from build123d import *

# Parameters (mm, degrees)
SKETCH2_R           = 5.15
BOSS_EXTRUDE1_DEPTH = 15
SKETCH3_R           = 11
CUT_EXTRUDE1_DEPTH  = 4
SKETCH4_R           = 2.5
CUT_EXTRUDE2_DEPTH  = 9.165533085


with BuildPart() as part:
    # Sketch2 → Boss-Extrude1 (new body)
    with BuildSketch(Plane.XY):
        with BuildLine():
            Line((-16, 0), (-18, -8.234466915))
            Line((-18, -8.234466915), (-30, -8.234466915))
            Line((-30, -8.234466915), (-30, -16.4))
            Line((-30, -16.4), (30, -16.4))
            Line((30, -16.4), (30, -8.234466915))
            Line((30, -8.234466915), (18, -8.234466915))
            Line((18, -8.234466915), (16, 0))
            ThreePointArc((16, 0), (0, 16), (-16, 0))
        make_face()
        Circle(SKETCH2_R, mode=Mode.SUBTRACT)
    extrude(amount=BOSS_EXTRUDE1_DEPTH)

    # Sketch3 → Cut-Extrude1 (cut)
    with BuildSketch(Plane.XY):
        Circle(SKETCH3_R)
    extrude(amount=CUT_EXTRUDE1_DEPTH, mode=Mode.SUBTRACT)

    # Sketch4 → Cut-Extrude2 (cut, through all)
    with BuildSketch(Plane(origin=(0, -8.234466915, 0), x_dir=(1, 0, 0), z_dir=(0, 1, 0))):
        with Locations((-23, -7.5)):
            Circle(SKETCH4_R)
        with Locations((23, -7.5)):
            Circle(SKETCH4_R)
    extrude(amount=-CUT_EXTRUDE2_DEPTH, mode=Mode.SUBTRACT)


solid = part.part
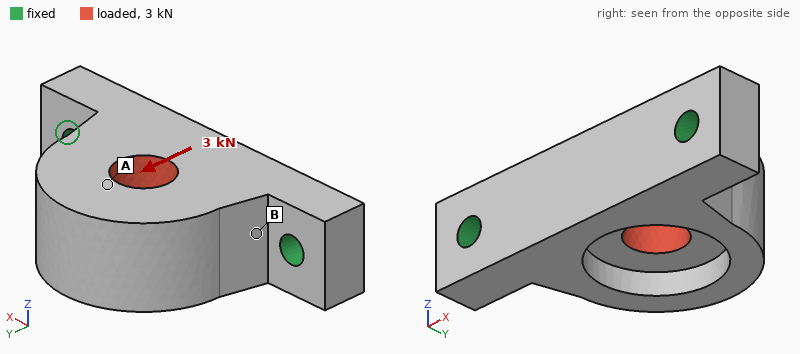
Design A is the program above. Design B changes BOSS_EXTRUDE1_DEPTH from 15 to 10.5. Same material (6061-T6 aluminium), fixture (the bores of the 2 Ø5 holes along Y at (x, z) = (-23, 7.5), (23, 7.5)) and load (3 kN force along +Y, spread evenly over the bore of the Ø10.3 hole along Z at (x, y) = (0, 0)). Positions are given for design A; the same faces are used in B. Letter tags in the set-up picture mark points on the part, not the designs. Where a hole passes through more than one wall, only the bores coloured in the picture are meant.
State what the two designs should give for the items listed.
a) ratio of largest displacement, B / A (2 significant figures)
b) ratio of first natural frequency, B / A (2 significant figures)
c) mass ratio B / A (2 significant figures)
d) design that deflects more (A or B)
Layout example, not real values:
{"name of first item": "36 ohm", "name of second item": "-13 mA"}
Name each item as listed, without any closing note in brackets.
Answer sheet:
{"ratio of largest displacement, B / A": "1.4", "ratio of first natural frequency, B / A": "0.88", "mass ratio B / A": "0.67", "design that deflects more": "B"}
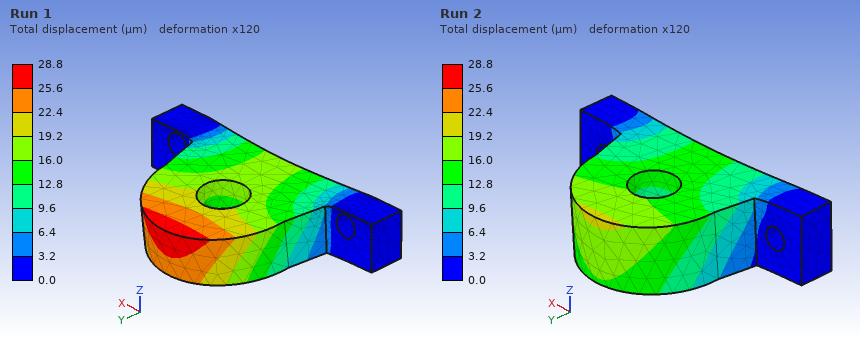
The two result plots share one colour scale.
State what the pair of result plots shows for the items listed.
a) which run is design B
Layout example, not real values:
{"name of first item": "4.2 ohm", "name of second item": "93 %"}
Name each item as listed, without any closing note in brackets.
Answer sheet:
{"which run is design B": "Run 1"}
